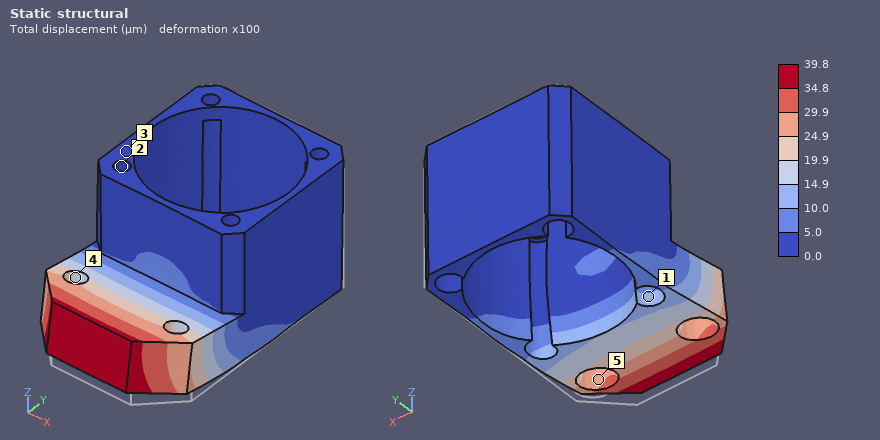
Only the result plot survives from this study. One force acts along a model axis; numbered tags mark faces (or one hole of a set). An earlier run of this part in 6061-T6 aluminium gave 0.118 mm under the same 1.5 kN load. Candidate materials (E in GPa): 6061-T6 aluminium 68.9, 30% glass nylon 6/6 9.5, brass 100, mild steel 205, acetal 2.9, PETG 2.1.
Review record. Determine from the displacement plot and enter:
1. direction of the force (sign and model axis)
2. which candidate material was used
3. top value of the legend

+Z
mild steel
39.8 µm
